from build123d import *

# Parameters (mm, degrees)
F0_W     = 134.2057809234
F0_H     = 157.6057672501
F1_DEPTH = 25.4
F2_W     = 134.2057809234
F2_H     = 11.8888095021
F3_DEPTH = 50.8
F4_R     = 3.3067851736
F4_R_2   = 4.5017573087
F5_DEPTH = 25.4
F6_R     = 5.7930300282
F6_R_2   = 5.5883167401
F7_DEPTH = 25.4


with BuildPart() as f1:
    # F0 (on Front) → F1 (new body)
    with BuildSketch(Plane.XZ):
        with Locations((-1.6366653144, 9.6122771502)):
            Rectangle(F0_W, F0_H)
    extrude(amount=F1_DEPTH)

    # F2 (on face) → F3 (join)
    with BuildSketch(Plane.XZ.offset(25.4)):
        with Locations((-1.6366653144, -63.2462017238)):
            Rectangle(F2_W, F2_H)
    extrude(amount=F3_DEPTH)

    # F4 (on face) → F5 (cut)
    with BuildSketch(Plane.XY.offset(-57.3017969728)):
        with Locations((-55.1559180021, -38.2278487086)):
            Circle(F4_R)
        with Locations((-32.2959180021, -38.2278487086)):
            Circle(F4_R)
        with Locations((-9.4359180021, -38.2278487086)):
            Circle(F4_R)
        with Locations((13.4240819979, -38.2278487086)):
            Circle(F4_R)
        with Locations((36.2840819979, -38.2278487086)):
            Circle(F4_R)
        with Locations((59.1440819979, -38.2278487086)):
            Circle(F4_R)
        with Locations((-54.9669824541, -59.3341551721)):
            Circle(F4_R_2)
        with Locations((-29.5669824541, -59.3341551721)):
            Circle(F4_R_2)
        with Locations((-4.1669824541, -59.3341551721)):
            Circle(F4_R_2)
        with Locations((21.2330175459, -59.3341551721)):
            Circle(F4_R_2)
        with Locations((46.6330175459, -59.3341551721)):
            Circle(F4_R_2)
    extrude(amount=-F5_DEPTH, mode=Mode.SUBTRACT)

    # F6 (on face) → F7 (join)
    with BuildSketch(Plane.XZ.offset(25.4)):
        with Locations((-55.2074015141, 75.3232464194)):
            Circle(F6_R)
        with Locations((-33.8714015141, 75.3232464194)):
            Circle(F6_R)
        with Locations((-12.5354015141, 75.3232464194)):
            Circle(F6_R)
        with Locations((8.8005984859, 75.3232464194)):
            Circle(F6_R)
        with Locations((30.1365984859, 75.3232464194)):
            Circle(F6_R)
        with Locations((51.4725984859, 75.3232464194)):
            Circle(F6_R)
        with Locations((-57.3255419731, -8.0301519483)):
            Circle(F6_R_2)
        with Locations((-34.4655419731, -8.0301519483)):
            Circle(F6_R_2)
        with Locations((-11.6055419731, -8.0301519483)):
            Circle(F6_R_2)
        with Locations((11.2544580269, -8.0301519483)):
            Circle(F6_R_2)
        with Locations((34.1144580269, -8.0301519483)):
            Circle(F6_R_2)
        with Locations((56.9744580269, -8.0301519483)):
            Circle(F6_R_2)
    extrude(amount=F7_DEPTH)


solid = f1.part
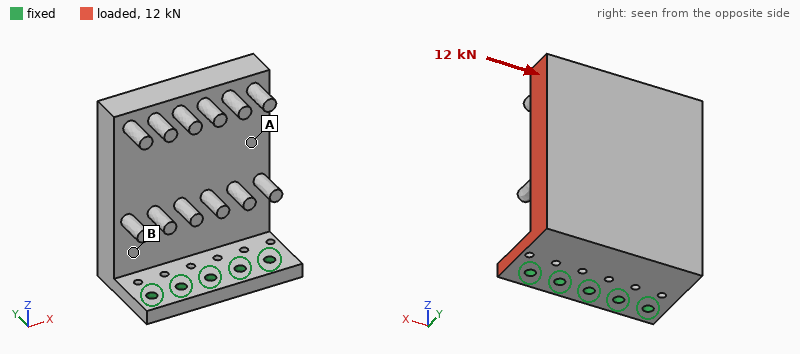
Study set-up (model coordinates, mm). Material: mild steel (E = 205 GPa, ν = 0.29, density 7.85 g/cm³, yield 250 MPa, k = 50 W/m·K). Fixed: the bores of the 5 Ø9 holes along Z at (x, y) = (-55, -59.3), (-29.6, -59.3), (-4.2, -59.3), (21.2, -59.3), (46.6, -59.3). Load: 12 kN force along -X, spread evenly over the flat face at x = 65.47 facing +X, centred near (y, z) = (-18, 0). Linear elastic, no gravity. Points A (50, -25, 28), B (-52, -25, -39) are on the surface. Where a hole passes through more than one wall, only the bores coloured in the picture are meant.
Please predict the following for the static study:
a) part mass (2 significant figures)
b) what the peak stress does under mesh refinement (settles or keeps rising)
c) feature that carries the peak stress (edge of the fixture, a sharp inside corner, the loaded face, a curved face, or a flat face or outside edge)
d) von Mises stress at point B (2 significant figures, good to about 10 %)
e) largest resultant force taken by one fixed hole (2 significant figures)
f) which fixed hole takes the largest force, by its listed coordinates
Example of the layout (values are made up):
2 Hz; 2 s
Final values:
5.0 kg; keeps rising; edge of the fixture; 28 MPa; 8.1 kN; (46.6, -59.3)
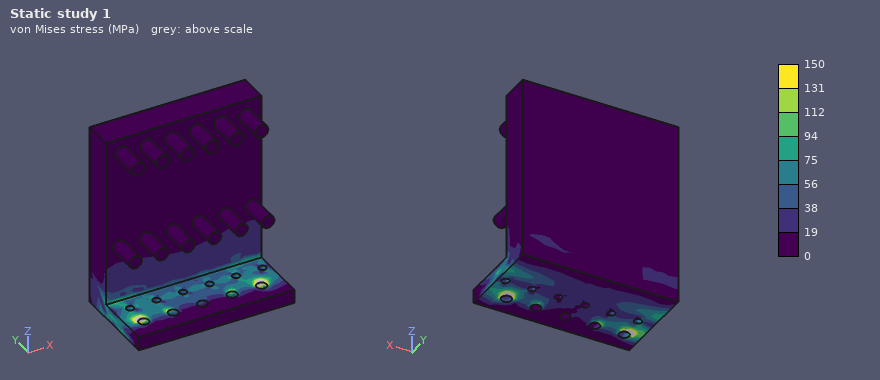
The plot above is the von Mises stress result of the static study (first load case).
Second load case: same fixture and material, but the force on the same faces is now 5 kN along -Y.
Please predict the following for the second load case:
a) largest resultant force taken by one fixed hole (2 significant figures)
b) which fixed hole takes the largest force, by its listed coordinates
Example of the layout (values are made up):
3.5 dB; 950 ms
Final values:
4.2 kN; (46.6, -59.3)
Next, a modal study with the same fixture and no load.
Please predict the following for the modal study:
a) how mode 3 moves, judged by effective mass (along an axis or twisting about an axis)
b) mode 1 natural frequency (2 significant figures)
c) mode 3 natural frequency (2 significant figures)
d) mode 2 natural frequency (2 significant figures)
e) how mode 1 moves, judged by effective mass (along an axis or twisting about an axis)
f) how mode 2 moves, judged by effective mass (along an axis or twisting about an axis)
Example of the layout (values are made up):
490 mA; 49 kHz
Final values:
along Z; 250 Hz; 1700 Hz; 700 Hz; along Y; along X
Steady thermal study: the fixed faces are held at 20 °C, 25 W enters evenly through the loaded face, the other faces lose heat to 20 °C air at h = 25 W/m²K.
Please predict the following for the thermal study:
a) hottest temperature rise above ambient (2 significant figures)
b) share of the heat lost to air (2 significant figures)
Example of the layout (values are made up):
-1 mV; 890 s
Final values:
13 K; 50 %
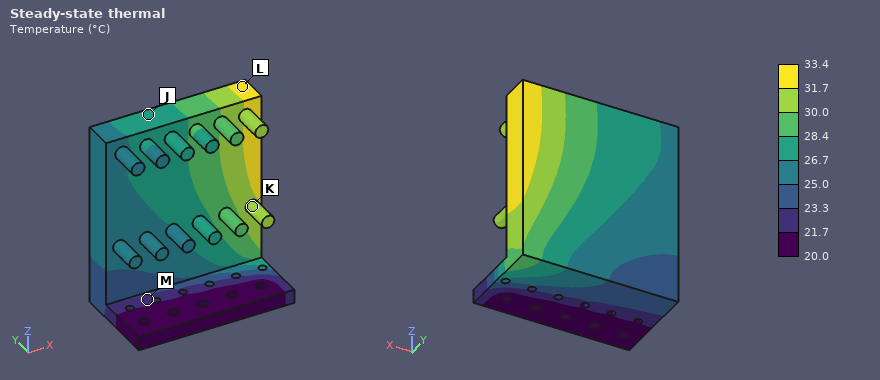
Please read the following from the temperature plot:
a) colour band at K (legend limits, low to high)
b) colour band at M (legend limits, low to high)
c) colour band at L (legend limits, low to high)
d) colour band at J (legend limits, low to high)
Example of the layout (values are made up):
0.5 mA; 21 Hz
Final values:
30.0 to 31.7 °C; 21.7 to 23.3 °C; 31.7 to 33.4 °C; 26.7 to 28.4 °C
